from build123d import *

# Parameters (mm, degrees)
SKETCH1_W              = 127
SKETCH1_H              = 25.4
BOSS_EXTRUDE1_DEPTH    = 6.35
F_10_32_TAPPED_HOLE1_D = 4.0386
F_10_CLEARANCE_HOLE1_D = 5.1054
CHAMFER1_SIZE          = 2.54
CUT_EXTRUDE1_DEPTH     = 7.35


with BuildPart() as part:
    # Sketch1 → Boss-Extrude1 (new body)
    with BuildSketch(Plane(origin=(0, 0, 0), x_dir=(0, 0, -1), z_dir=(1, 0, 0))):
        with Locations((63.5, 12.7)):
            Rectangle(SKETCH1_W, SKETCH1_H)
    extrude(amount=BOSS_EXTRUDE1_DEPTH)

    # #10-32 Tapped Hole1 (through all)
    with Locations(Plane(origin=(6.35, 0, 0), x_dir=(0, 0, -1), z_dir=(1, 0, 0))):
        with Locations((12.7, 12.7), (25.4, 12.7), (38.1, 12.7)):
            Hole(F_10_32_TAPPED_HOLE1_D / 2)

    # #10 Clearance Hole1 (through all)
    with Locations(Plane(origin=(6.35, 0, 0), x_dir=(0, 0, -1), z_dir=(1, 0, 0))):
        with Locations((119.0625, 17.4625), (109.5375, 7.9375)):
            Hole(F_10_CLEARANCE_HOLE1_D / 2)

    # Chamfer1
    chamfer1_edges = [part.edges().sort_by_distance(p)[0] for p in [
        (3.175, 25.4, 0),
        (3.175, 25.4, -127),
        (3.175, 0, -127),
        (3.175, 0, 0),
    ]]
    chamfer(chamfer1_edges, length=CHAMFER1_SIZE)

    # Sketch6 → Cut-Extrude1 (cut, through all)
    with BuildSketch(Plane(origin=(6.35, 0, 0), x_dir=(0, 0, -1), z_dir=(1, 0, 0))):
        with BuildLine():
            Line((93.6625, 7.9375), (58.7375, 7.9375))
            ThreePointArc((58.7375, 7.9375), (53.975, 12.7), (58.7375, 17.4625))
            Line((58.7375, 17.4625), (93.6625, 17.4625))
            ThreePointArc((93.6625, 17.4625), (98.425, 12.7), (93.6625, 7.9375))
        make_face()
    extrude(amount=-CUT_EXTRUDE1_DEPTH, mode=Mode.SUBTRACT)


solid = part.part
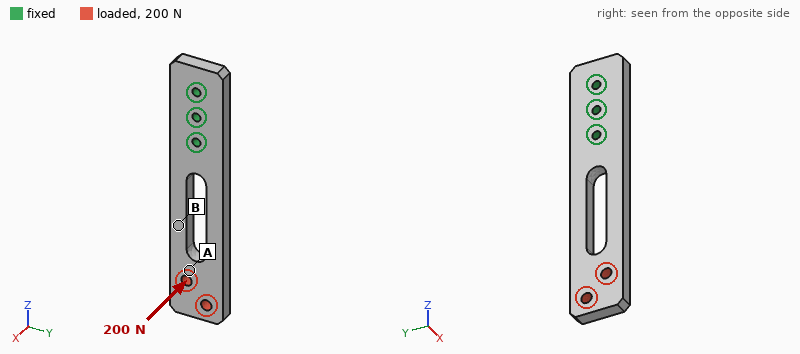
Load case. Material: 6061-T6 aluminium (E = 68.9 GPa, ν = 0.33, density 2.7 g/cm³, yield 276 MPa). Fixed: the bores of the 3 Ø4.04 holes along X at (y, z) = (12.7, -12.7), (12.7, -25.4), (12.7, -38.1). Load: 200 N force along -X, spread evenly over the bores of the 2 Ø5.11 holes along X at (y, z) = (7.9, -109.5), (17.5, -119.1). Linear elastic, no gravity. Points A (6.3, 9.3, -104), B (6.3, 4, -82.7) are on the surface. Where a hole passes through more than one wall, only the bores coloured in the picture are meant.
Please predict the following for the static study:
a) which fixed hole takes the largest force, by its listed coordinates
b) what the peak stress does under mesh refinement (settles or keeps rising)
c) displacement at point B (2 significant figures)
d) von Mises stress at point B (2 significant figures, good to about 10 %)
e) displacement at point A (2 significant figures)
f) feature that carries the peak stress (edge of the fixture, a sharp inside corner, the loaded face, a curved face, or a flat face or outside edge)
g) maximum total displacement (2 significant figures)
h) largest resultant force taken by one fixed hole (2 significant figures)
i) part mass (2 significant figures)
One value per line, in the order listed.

(12.7, -38.1)
keeps rising
0.42 mm
59 MPa
0.84 mm
edge of the fixture
1.3 mm
660 N
47 g
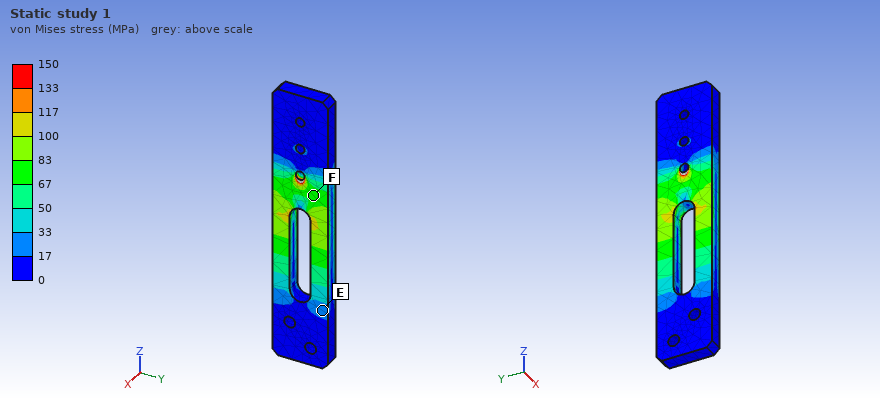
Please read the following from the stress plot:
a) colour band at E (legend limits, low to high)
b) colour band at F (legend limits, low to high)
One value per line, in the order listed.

17 to 33 MPa
67 to 83 MPa
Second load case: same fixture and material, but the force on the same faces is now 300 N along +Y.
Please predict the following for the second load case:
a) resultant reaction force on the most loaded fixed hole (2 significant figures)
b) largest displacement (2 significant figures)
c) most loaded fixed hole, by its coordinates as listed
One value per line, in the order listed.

1.2 kN
0.21 mm
(12.7, -38.1)
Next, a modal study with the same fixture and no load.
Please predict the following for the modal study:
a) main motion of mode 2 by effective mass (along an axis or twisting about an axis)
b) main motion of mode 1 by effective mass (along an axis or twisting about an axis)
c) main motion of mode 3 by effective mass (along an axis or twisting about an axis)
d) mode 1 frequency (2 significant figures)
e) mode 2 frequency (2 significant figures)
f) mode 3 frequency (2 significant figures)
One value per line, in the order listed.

along Y
along X
twisting about Z
610 Hz
1700 Hz
3000 Hz
